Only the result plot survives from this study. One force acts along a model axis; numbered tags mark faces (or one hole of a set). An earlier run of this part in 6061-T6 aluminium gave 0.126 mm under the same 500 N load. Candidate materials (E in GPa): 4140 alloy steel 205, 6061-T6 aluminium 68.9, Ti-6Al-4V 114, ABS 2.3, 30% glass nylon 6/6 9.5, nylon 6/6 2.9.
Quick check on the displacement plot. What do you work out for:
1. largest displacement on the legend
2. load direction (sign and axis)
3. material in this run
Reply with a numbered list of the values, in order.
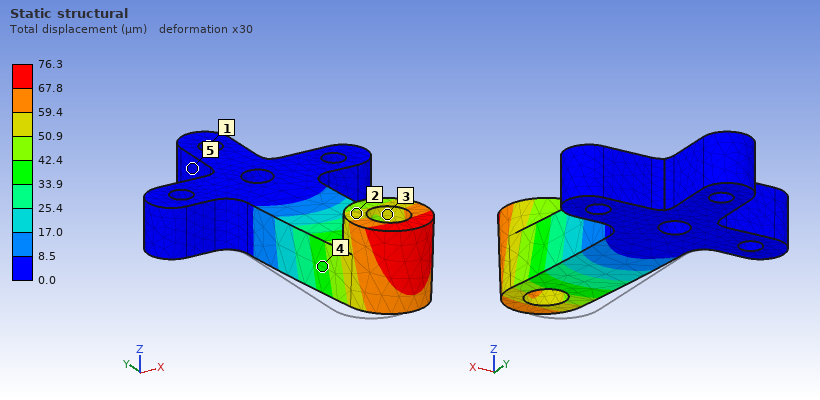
1. 76.3 µm
2. +X
3. Ti-6Al-4V
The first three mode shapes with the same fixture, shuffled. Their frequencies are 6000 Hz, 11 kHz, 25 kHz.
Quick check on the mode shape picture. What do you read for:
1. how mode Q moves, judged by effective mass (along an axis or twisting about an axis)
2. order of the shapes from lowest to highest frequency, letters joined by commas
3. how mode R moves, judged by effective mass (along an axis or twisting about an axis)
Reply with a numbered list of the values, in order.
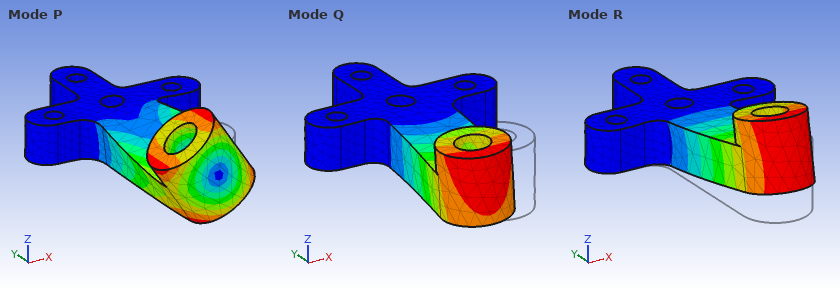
1. along X
2. R, Q, P
3. along Z
